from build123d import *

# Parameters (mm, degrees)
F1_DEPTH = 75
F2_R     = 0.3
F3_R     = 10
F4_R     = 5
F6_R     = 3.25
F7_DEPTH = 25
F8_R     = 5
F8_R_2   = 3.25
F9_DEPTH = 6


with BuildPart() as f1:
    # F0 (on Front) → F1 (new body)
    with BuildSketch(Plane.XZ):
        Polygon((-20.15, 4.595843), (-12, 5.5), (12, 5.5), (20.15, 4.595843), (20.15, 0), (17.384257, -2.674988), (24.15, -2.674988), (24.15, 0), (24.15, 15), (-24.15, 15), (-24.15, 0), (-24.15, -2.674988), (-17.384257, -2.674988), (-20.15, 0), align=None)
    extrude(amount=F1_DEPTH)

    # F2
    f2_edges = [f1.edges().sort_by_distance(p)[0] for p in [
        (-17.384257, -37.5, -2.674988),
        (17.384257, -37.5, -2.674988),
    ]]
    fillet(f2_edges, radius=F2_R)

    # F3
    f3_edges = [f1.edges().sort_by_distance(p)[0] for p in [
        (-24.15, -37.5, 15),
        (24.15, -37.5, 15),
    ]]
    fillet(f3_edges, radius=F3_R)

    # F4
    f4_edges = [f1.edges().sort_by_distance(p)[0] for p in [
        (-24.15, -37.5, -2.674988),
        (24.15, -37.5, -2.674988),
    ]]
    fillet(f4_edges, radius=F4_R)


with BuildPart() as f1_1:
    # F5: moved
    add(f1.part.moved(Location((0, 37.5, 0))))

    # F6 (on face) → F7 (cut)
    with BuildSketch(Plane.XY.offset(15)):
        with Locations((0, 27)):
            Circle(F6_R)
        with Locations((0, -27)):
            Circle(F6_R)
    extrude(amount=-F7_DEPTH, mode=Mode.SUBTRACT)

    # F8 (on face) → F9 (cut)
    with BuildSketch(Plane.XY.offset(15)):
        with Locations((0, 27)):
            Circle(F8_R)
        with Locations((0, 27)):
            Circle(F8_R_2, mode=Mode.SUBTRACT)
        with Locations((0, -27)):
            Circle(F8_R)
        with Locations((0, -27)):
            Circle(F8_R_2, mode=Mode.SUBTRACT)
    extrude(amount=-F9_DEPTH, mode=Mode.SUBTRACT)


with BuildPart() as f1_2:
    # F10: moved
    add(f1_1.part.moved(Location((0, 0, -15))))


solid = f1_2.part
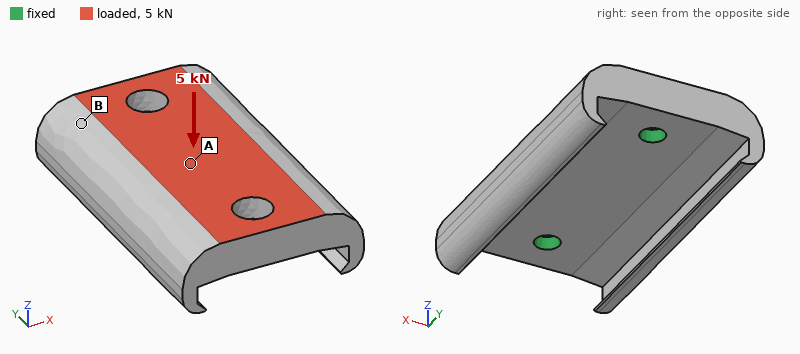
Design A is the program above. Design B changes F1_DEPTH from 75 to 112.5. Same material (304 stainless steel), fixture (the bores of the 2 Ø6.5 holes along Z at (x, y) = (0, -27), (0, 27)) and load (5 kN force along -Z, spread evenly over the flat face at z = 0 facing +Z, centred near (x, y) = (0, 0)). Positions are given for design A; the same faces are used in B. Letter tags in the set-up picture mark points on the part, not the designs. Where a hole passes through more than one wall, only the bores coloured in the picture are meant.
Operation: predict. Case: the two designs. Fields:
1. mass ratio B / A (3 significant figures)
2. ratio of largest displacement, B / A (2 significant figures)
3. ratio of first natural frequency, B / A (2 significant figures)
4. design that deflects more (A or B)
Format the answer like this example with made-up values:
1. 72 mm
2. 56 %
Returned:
1. 1.52
2. 7.4
3. 0.75
4. B
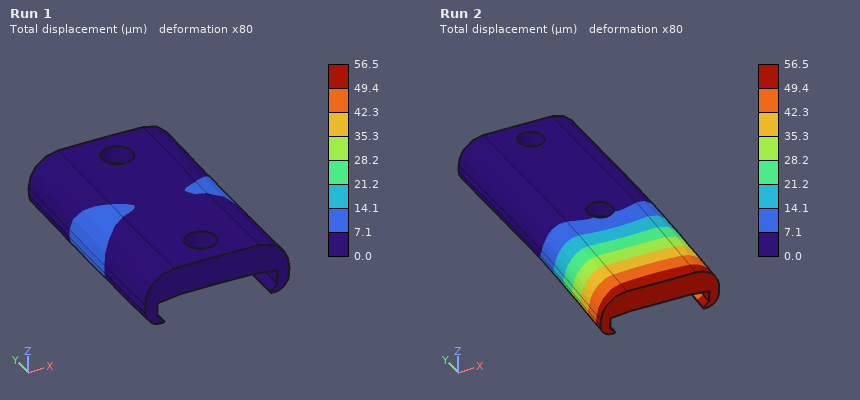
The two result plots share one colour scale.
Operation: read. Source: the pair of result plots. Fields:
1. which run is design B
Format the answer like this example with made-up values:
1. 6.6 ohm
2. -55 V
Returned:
1. Run 2
